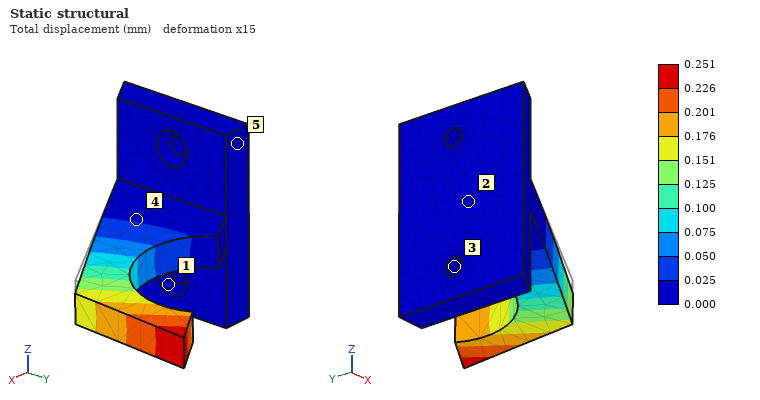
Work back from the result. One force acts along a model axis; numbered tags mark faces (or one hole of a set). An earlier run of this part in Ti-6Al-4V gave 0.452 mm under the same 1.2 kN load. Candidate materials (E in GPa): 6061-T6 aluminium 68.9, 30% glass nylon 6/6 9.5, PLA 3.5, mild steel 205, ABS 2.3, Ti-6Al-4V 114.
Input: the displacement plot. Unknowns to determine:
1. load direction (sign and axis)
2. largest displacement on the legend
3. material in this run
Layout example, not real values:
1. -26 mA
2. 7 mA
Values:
1. -Z
2. 0.251 mm
3. mild steel
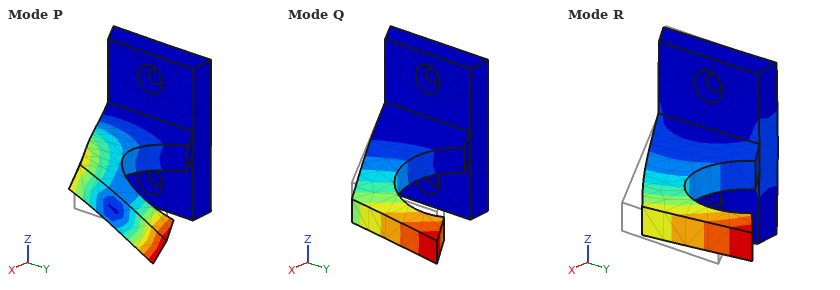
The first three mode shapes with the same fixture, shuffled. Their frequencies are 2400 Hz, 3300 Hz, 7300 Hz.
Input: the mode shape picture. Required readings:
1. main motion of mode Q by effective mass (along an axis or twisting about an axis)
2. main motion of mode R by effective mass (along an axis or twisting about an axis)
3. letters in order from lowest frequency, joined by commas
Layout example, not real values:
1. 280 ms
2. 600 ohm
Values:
1. along Z
2. along Y
3. Q, R, P
